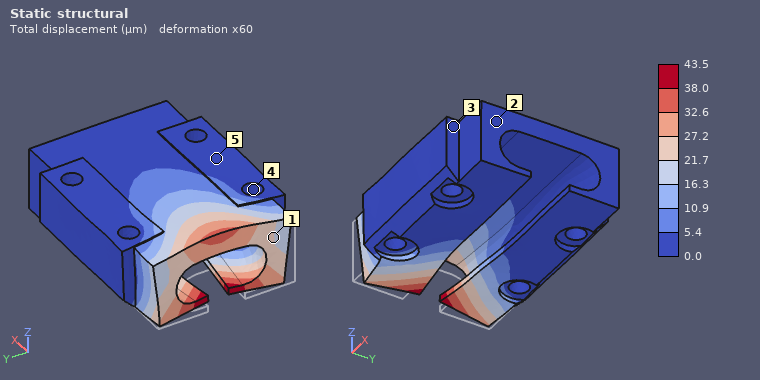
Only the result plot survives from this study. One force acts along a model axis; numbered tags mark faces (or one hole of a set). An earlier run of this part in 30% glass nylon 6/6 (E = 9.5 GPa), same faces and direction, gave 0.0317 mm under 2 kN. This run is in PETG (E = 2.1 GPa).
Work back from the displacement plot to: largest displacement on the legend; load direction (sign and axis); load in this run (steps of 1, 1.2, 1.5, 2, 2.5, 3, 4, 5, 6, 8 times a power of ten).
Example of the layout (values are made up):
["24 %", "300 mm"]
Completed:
["43.5 µm", "+X", "600 N"]
